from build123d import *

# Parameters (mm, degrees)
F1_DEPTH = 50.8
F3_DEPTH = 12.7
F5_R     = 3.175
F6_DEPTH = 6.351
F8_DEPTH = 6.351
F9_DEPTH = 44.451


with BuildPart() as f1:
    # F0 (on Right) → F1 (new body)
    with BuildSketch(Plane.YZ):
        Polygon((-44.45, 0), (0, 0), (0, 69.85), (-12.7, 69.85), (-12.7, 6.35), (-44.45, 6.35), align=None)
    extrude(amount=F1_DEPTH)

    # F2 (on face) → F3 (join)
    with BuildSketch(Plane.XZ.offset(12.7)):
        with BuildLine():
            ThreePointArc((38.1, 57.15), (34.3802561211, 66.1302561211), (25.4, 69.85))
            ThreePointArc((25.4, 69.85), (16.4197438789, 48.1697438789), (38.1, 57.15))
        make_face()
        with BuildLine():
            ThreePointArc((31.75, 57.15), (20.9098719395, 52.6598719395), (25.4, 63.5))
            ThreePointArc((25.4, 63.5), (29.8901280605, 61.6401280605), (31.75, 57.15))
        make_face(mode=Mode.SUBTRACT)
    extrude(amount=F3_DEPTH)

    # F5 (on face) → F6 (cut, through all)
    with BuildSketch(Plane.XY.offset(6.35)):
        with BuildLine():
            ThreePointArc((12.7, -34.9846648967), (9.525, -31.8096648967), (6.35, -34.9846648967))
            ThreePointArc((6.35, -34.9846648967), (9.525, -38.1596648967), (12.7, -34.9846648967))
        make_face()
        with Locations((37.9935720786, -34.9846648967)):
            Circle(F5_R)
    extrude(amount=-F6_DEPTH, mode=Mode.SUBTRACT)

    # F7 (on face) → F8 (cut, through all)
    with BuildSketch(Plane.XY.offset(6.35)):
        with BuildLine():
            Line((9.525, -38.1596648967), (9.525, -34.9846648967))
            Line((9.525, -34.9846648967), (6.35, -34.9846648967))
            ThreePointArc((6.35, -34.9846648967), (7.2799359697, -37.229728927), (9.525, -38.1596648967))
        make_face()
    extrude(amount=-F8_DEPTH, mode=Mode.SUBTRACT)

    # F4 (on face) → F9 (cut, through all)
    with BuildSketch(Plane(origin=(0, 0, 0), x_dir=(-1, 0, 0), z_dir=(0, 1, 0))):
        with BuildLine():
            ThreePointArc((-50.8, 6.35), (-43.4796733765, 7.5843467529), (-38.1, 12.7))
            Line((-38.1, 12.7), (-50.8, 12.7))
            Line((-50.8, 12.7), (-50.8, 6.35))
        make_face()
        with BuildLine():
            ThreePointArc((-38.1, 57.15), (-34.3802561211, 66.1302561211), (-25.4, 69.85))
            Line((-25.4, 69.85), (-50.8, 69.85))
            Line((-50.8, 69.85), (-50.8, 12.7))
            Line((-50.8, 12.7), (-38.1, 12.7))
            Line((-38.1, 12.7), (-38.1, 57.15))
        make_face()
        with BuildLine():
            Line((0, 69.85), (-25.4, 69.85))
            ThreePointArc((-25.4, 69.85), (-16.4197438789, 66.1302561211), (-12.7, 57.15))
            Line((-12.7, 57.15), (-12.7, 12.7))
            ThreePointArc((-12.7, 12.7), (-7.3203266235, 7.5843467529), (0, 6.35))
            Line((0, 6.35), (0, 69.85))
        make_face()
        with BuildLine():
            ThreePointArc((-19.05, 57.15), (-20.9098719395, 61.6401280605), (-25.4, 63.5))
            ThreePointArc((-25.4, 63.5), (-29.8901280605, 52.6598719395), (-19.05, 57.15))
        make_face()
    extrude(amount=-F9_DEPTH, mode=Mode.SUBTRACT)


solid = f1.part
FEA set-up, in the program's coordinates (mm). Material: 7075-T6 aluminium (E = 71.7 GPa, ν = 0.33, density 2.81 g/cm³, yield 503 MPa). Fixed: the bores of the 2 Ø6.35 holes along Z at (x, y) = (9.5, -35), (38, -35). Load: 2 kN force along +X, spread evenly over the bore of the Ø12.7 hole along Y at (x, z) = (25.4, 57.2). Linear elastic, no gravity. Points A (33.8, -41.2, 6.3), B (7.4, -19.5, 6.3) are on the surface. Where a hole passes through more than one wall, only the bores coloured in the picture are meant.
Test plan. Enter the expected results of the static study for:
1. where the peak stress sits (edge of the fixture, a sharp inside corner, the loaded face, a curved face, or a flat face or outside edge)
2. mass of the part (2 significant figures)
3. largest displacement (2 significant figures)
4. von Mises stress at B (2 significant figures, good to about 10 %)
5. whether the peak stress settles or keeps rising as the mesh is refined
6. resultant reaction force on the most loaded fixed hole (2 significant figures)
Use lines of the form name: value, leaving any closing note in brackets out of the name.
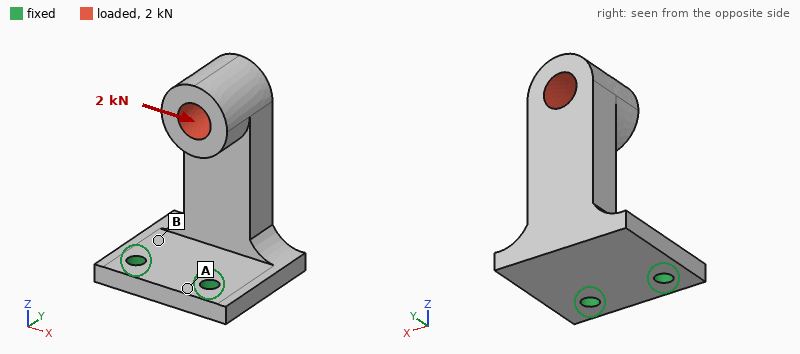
where the peak stress sits: edge of the fixture
mass of the part: 100 g
largest displacement: 0.83 mm
von Mises stress at B: 120 MPa
whether the peak stress settles or keeps rising as the mesh is refined: keeps rising
resultant reaction force on the most loaded fixed hole: 3.6 kN
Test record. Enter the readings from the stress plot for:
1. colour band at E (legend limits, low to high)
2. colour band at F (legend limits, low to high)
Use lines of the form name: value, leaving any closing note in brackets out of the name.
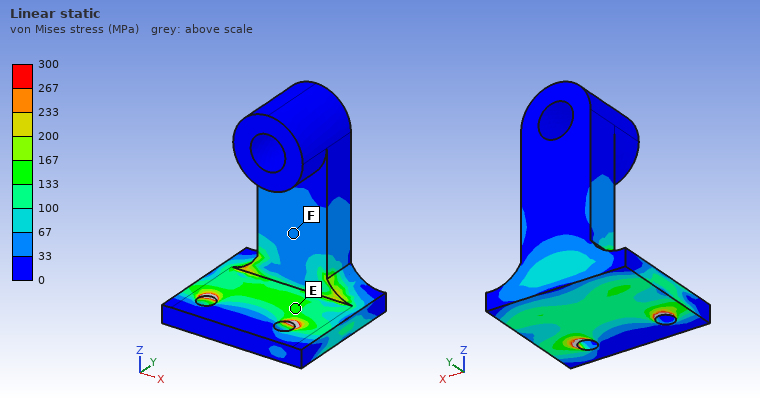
colour band at E: 133 to 167 MPa
colour band at F: 33 to 67 MPa
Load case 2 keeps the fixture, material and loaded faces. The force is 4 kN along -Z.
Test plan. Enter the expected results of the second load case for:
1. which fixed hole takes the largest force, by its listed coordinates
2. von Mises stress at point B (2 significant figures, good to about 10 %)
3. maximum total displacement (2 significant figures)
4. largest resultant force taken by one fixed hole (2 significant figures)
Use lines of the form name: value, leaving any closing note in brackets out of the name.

which fixed hole takes the largest force, by its listed coordinates: (38, -35)
von Mises stress at point B: 79 MPa
maximum total displacement: 0.70 mm
largest resultant force taken by one fixed hole: 2.2 kN
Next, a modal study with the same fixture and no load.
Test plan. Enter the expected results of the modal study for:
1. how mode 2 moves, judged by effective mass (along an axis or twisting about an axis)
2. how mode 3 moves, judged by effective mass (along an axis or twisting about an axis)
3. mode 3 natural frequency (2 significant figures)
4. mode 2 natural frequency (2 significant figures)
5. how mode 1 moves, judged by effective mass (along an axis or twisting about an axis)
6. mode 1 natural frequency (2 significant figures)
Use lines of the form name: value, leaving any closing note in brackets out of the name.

how mode 2 moves, judged by effective mass: along X
how mode 3 moves, judged by effective mass: along Z
mode 3 natural frequency: 3200 Hz
mode 2 natural frequency: 1500 Hz
how mode 1 moves, judged by effective mass: along Y
mode 1 natural frequency: 770 Hz
